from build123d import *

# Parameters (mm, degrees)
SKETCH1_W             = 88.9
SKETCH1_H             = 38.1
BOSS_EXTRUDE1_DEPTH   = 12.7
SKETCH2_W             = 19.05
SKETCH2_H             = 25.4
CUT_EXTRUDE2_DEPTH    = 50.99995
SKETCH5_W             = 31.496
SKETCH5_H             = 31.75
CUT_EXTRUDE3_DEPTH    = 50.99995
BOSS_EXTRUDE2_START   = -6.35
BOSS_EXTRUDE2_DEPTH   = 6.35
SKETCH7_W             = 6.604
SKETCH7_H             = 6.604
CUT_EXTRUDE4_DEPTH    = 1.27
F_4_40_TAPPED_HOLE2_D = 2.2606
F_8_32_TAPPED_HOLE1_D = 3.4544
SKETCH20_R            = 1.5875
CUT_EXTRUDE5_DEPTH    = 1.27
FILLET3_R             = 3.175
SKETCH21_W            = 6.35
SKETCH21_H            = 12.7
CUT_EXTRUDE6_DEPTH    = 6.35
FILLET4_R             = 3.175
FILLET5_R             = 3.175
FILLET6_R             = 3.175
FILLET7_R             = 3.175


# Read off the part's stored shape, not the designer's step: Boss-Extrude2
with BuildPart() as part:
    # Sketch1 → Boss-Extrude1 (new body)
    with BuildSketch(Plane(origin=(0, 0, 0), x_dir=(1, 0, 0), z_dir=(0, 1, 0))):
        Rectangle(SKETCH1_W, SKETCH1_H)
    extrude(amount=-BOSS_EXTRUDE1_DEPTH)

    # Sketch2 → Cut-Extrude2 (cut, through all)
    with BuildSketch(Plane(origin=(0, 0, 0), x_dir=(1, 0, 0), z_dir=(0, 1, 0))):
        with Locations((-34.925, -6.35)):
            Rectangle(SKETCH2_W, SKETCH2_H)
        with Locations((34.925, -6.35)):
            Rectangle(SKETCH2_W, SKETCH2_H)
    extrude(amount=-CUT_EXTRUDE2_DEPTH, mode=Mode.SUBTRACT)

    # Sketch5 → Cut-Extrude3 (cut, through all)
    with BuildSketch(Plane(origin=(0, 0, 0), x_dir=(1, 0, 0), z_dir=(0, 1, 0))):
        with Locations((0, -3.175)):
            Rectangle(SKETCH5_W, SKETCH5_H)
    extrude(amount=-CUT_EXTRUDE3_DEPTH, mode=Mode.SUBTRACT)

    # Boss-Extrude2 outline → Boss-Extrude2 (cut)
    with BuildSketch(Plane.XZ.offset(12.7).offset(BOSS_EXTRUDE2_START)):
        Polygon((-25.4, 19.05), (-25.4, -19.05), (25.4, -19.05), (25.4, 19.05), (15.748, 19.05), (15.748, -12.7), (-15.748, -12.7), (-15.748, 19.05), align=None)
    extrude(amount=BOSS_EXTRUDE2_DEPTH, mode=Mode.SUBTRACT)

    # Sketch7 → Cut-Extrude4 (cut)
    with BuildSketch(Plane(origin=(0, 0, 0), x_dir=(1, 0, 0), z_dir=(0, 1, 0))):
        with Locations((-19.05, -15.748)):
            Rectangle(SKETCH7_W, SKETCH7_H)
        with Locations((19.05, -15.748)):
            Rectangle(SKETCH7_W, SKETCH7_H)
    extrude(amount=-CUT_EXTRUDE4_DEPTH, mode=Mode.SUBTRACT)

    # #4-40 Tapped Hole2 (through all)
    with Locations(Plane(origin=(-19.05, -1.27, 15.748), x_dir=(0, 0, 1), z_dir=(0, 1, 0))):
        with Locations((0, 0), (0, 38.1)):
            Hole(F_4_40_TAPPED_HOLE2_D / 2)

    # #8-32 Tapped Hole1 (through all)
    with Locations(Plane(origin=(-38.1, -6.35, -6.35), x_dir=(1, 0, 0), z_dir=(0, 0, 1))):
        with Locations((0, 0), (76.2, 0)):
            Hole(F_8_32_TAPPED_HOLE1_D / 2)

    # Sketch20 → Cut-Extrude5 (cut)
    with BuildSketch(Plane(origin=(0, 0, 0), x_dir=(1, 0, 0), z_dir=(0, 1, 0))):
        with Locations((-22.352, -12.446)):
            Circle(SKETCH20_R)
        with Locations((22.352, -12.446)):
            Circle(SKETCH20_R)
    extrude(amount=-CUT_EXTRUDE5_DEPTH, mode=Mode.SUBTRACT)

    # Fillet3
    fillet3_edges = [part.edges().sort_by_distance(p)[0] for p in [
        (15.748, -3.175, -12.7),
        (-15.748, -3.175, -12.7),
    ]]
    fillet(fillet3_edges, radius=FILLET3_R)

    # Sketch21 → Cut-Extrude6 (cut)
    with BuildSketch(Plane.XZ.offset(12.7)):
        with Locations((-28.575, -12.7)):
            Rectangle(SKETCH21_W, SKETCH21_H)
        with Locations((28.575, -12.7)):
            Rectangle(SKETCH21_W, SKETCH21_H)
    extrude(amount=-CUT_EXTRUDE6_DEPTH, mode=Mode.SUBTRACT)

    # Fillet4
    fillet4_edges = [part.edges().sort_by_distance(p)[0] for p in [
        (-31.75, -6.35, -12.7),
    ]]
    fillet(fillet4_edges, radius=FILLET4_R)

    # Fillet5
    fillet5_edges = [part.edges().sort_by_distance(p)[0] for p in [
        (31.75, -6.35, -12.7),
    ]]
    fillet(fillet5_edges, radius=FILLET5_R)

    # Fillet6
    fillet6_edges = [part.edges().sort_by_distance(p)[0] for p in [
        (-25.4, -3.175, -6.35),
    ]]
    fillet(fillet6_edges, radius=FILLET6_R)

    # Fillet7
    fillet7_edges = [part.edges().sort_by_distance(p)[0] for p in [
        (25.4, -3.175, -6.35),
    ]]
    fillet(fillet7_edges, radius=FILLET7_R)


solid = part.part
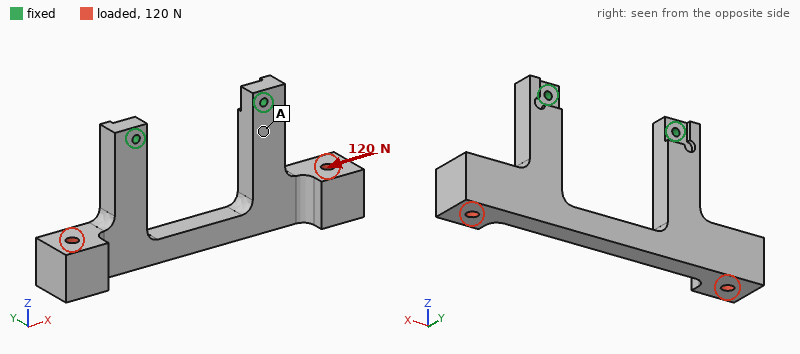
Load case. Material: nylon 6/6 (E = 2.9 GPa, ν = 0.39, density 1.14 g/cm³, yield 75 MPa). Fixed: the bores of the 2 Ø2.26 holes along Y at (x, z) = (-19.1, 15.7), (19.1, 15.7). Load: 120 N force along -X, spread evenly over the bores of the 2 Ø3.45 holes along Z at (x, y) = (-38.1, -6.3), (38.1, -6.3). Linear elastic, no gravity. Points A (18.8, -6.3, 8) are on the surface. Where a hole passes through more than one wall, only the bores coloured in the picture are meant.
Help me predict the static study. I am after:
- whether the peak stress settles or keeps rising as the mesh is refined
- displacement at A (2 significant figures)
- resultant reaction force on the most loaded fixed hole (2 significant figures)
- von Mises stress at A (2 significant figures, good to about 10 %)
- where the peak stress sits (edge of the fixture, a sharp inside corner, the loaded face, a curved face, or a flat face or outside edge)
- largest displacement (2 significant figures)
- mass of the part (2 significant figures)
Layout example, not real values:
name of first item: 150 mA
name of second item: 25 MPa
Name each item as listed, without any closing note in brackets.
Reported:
whether the peak stress settles or keeps rising as the mesh is refined: keeps rising
displacement at A: 0.11 mm
resultant reaction force on the most loaded fixed hole: 74 N
von Mises stress at A: 5.1 MPa
where the peak stress sits: edge of the fixture
largest displacement: 0.67 mm
mass of the part: 12 g
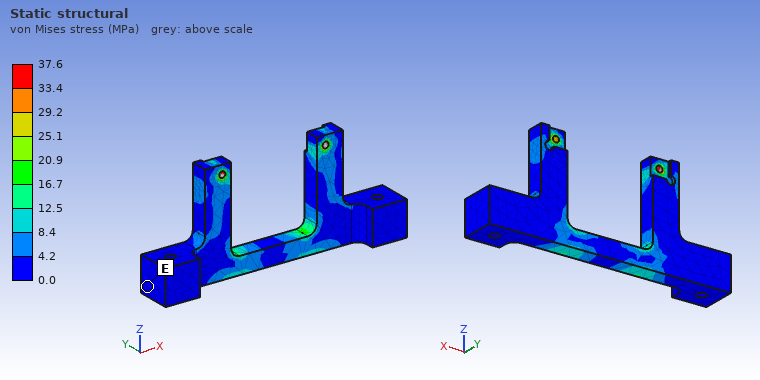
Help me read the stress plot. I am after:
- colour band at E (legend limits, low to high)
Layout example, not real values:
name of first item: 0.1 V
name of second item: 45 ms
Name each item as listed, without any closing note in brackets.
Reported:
colour band at E: 0.0 to 4.2 MPa
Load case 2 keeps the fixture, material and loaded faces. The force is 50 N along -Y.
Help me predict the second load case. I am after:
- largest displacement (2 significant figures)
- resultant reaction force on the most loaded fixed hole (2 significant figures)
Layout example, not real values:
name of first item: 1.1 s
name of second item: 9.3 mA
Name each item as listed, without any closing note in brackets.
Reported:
largest displacement: 1.0 mm
resultant reaction force on the most loaded fixed hole: 25 N
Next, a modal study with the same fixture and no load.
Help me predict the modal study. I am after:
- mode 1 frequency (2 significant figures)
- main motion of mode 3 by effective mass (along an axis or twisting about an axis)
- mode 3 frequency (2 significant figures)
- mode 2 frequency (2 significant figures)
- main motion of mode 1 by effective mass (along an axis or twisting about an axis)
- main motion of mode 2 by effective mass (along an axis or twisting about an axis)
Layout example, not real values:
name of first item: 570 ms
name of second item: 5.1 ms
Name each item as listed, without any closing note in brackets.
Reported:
mode 1 frequency: 480 Hz
main motion of mode 3 by effective mass: along X
mode 3 frequency: 810 Hz
mode 2 frequency: 510 Hz
main motion of mode 1 by effective mass: along Y
main motion of mode 2 by effective mass: twisting about Z
